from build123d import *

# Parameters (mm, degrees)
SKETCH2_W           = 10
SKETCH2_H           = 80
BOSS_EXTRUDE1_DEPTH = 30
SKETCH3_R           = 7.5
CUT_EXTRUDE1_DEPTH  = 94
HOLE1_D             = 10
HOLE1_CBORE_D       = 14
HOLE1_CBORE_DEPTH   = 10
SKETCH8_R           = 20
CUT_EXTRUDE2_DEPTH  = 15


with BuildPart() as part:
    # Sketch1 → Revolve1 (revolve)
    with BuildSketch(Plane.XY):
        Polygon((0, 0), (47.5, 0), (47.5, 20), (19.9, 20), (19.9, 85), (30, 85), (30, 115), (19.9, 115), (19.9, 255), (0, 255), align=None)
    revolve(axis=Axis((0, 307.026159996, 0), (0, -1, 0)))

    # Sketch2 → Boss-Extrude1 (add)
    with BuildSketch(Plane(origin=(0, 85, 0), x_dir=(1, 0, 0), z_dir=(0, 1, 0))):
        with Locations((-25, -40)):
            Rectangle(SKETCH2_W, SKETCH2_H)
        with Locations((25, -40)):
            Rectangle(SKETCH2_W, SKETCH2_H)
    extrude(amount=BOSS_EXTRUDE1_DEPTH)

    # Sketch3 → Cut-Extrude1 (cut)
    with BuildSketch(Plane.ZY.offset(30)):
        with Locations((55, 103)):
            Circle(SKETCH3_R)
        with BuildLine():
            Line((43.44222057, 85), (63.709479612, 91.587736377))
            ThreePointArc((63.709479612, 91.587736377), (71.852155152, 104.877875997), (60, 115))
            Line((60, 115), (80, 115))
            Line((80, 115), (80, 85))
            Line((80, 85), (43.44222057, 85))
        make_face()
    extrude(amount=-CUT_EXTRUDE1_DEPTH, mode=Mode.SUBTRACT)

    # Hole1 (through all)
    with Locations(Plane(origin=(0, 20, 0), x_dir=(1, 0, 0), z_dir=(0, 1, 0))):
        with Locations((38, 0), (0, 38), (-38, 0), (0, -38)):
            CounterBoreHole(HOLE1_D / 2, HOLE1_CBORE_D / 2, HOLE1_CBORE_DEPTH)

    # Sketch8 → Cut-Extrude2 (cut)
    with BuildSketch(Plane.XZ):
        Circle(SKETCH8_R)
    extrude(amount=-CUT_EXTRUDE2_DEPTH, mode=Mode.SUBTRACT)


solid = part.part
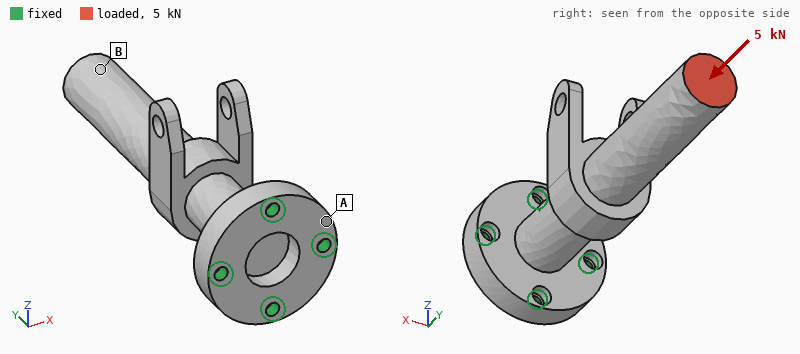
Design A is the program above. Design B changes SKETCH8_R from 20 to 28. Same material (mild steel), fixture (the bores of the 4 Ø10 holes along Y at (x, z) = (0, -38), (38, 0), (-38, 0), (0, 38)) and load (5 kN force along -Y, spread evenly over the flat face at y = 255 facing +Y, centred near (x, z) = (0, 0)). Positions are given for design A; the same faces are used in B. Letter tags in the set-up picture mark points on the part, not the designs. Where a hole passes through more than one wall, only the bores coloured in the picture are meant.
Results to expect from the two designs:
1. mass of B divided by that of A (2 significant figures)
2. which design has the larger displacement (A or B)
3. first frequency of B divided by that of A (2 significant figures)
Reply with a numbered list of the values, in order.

1. 0.96
2. B
3. 0.82
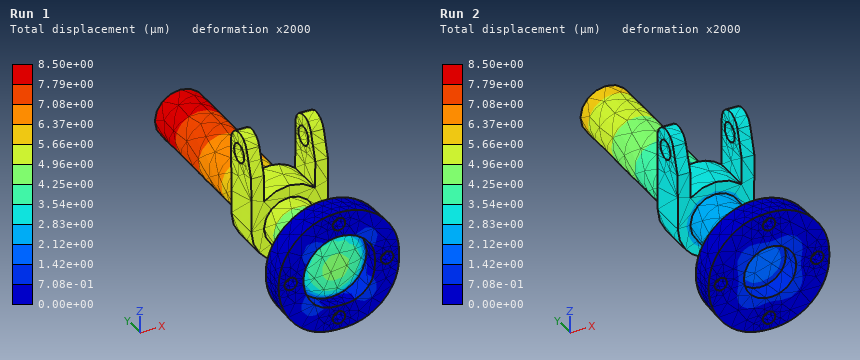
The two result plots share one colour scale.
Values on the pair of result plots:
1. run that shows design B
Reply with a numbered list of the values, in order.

1. Run 1
